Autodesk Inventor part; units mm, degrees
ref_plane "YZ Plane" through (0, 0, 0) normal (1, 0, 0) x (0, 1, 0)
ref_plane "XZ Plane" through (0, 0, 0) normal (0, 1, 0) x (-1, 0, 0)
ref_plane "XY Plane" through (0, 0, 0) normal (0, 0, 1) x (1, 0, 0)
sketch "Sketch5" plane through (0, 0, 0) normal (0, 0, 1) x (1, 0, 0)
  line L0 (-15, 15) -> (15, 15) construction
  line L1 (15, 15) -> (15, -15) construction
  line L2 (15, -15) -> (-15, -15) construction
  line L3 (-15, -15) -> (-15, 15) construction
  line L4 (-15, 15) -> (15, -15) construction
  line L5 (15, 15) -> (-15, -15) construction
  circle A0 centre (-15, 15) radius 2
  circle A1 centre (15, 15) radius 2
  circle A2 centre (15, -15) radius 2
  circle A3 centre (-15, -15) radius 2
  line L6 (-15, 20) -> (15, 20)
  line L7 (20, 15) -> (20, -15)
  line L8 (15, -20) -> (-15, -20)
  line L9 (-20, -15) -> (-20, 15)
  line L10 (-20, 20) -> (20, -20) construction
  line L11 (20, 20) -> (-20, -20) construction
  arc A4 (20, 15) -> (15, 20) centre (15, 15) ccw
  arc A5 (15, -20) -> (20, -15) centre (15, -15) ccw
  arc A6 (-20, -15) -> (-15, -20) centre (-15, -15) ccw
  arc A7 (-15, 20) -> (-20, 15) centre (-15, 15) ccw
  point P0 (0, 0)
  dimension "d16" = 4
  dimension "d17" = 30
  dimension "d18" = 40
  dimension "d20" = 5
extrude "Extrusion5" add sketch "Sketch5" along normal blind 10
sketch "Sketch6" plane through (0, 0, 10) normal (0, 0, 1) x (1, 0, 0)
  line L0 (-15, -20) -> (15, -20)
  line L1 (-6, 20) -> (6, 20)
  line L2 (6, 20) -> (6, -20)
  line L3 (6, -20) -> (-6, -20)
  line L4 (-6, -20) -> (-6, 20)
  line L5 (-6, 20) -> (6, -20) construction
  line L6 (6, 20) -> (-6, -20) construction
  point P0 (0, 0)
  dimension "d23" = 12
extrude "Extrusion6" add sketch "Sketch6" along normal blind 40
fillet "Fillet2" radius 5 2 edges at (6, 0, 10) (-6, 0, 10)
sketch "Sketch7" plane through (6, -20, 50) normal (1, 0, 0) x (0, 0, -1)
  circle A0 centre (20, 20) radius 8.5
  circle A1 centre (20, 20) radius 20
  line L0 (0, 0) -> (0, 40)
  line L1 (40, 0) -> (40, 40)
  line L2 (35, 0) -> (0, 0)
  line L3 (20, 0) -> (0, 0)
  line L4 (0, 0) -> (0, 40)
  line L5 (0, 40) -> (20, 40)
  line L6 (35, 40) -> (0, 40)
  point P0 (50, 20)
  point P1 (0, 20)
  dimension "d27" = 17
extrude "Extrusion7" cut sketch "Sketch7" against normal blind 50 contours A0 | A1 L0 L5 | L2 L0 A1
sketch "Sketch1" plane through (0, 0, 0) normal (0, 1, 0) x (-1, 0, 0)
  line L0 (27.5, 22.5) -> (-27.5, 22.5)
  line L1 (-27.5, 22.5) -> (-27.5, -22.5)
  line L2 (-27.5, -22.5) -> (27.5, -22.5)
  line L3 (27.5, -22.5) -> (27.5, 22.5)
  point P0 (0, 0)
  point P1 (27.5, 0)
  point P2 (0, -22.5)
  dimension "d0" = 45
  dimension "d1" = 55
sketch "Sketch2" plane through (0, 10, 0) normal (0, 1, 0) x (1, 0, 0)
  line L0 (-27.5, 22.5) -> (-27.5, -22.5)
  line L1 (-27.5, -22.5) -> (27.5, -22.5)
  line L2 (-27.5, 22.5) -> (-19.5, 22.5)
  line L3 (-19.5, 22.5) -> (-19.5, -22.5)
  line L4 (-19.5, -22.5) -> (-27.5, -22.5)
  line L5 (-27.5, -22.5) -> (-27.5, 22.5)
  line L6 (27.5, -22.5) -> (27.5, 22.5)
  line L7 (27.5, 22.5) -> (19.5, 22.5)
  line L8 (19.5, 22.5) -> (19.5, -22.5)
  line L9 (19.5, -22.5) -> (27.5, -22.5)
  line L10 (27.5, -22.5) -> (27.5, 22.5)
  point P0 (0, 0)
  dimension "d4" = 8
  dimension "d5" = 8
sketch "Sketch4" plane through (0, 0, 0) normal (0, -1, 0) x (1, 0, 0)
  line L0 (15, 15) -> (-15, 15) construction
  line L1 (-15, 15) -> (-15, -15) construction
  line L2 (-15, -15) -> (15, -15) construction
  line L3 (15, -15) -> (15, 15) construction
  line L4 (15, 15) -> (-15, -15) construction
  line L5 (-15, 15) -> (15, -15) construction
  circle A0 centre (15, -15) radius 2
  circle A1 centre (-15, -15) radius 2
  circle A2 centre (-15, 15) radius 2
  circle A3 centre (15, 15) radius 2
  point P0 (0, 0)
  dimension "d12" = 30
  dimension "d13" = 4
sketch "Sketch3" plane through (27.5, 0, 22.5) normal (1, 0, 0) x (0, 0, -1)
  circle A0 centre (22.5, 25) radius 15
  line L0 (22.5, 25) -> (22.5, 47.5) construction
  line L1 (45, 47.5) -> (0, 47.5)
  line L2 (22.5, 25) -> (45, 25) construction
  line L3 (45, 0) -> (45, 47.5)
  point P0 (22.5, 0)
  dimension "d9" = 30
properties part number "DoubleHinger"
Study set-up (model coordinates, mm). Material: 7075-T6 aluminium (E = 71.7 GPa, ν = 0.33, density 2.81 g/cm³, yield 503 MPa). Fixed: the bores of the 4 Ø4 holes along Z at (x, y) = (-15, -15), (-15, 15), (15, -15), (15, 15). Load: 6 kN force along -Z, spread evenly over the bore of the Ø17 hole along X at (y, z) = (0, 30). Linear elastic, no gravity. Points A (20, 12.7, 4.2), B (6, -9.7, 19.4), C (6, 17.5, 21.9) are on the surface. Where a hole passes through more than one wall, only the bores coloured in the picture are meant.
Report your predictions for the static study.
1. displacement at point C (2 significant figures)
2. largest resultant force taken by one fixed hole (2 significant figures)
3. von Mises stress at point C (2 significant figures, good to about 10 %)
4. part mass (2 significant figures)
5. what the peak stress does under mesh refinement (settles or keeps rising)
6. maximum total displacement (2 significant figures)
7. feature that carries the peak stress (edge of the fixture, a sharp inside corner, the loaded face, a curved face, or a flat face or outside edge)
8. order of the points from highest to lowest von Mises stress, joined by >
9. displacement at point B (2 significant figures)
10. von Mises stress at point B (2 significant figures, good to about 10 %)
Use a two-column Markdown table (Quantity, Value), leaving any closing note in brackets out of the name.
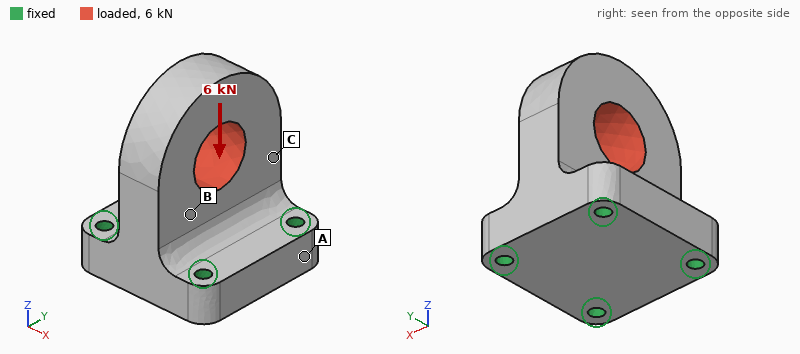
| Quantity | Value |
|---|---|
| displacement at point C | 7.9 µm |
| largest resultant force taken by one fixed hole | 1.6 kN |
| von Mises stress at point C | 11 MPa |
| part mass | 85 g |
| what the peak stress does under mesh refinement | keeps rising |
| maximum total displacement | 15 µm |
| feature that carries the peak stress | edge of the fixture |
| order of the points from highest to lowest von Mises stress, joined by > | B > C > A |
| displacement at point B | 7.3 µm |
| von Mises stress at point B | 17 MPa |
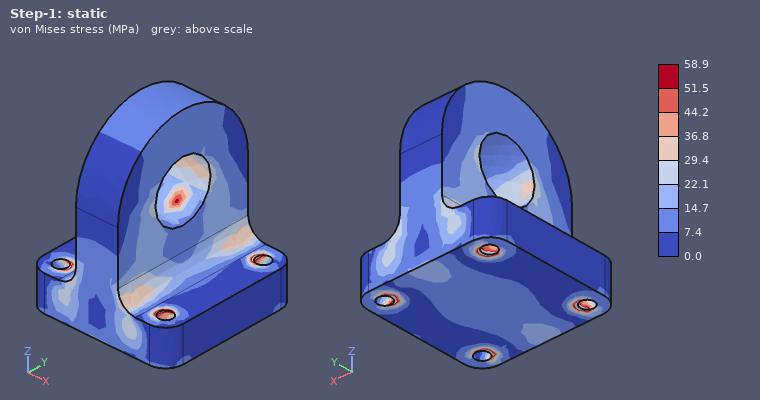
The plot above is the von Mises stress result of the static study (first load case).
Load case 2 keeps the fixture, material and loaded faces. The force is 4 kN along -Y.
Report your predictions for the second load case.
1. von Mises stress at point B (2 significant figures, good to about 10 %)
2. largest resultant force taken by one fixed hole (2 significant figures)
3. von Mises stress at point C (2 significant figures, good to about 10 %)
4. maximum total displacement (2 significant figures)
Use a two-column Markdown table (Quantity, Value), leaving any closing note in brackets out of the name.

| Quantity | Value |
|---|---|
| von Mises stress at point B | 12 MPa |
| largest resultant force taken by one fixed hole | 2.0 kN |
| von Mises stress at point C | 16 MPa |
| maximum total displacement | 43 µm |
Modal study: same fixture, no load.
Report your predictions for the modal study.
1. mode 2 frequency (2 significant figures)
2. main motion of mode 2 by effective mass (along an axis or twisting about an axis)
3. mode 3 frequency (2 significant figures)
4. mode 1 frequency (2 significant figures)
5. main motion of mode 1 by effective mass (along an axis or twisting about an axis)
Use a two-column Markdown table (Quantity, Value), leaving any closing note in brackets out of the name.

| Quantity | Value |
|---|---|
| mode 2 frequency | 9100 Hz |
| main motion of mode 2 by effective mass | along Y |
| mode 3 frequency | 13 kHz |
| mode 1 frequency | 6000 Hz |
| main motion of mode 1 by effective mass | along X |
